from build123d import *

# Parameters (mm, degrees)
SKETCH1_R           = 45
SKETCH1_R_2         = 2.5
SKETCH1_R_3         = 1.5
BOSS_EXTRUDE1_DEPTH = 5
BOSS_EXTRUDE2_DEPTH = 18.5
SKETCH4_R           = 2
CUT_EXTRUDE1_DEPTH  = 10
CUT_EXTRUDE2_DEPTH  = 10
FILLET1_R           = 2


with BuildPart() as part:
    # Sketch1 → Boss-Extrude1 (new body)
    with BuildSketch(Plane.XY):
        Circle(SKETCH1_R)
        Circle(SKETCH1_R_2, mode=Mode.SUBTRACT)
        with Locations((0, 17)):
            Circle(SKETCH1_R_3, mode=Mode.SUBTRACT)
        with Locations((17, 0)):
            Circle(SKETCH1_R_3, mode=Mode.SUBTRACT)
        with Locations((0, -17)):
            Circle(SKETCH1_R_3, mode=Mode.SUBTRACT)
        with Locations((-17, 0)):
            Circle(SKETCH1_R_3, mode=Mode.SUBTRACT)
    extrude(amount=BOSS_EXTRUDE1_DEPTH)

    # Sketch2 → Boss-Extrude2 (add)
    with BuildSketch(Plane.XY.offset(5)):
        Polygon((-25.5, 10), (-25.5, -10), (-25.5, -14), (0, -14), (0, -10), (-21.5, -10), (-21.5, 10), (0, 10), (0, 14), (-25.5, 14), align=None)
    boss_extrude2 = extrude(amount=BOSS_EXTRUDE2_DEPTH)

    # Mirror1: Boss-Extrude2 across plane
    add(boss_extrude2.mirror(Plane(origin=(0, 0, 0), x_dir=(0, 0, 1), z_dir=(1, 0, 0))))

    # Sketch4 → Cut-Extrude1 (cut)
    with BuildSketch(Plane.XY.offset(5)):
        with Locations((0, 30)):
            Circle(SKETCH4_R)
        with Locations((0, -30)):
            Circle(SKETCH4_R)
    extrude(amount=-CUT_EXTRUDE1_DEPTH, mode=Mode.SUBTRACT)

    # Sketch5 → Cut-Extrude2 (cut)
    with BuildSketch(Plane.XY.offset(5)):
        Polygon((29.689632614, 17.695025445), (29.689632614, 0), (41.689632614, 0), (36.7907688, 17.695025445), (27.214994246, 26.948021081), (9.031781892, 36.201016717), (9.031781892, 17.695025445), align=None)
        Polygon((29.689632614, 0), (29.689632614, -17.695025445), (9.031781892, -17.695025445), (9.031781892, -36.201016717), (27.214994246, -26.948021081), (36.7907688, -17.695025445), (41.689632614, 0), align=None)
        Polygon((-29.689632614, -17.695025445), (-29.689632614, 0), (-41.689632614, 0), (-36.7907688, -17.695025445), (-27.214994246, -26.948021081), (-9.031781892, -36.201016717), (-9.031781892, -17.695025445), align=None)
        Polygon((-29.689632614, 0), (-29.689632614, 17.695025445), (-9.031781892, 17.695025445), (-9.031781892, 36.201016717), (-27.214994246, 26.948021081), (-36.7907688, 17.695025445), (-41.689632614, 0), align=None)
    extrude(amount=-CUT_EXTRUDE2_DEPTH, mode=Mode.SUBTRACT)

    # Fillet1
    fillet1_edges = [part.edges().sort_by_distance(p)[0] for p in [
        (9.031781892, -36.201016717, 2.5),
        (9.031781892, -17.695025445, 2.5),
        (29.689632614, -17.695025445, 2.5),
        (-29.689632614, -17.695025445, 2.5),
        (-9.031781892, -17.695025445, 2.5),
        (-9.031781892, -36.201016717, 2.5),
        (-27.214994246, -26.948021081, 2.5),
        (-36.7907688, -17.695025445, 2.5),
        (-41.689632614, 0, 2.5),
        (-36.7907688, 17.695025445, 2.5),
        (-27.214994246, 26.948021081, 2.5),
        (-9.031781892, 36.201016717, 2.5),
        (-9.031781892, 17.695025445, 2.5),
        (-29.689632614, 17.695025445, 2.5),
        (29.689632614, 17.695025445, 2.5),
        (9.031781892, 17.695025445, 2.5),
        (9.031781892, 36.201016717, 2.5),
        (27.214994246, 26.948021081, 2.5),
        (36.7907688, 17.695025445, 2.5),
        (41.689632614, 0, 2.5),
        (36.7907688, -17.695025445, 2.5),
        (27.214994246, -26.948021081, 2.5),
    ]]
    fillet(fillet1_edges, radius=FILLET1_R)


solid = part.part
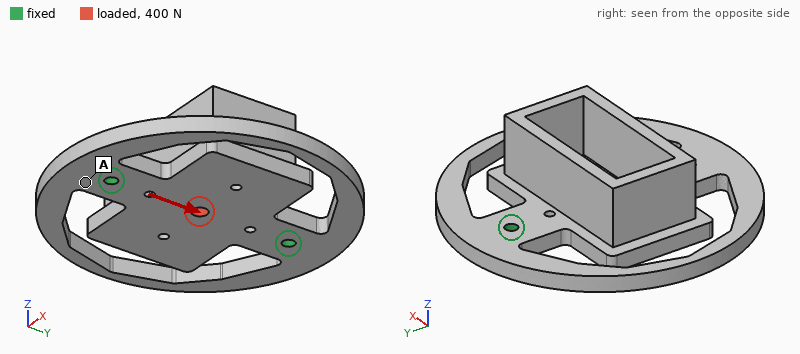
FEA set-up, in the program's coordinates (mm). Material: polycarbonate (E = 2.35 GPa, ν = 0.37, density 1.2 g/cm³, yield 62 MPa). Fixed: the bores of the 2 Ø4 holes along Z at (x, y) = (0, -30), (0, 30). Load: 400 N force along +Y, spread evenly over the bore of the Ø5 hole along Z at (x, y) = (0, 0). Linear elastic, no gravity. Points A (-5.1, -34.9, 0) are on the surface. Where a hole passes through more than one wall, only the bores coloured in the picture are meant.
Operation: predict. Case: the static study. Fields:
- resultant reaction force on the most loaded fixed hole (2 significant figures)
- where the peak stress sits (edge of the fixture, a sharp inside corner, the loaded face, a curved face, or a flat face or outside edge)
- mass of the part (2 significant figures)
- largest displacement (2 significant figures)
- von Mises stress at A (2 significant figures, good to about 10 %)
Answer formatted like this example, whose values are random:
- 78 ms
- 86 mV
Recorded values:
- 200 N
- the loaded face
- 39 g
- 36 µm
- 0.86 MPa
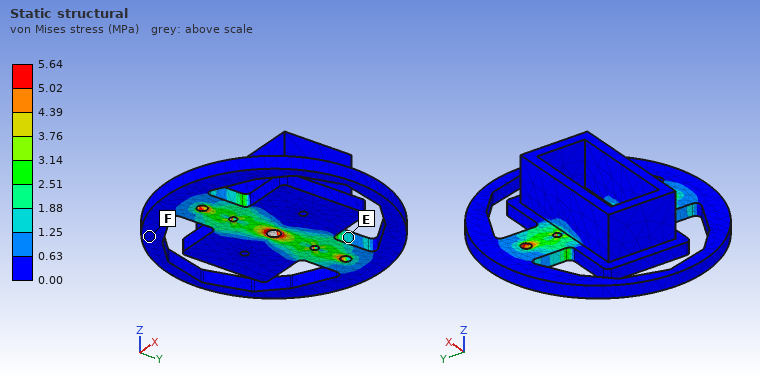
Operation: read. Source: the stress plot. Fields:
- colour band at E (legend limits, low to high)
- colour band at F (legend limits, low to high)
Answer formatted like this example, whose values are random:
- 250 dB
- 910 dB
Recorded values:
- 1.25 to 1.88 MPa
- 0.00 to 0.63 MPa
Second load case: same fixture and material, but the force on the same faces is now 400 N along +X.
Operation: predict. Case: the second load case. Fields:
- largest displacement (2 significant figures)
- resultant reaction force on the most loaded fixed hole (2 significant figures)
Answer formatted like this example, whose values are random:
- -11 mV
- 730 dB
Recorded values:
- 0.10 mm
- 200 N
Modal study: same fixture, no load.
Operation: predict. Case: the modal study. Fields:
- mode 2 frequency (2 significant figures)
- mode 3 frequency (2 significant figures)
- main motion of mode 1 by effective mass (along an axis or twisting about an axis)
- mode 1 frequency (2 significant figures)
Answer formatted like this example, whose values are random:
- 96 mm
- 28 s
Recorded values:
- 470 Hz
- 470 Hz
- twisting about Y
- 440 Hz
